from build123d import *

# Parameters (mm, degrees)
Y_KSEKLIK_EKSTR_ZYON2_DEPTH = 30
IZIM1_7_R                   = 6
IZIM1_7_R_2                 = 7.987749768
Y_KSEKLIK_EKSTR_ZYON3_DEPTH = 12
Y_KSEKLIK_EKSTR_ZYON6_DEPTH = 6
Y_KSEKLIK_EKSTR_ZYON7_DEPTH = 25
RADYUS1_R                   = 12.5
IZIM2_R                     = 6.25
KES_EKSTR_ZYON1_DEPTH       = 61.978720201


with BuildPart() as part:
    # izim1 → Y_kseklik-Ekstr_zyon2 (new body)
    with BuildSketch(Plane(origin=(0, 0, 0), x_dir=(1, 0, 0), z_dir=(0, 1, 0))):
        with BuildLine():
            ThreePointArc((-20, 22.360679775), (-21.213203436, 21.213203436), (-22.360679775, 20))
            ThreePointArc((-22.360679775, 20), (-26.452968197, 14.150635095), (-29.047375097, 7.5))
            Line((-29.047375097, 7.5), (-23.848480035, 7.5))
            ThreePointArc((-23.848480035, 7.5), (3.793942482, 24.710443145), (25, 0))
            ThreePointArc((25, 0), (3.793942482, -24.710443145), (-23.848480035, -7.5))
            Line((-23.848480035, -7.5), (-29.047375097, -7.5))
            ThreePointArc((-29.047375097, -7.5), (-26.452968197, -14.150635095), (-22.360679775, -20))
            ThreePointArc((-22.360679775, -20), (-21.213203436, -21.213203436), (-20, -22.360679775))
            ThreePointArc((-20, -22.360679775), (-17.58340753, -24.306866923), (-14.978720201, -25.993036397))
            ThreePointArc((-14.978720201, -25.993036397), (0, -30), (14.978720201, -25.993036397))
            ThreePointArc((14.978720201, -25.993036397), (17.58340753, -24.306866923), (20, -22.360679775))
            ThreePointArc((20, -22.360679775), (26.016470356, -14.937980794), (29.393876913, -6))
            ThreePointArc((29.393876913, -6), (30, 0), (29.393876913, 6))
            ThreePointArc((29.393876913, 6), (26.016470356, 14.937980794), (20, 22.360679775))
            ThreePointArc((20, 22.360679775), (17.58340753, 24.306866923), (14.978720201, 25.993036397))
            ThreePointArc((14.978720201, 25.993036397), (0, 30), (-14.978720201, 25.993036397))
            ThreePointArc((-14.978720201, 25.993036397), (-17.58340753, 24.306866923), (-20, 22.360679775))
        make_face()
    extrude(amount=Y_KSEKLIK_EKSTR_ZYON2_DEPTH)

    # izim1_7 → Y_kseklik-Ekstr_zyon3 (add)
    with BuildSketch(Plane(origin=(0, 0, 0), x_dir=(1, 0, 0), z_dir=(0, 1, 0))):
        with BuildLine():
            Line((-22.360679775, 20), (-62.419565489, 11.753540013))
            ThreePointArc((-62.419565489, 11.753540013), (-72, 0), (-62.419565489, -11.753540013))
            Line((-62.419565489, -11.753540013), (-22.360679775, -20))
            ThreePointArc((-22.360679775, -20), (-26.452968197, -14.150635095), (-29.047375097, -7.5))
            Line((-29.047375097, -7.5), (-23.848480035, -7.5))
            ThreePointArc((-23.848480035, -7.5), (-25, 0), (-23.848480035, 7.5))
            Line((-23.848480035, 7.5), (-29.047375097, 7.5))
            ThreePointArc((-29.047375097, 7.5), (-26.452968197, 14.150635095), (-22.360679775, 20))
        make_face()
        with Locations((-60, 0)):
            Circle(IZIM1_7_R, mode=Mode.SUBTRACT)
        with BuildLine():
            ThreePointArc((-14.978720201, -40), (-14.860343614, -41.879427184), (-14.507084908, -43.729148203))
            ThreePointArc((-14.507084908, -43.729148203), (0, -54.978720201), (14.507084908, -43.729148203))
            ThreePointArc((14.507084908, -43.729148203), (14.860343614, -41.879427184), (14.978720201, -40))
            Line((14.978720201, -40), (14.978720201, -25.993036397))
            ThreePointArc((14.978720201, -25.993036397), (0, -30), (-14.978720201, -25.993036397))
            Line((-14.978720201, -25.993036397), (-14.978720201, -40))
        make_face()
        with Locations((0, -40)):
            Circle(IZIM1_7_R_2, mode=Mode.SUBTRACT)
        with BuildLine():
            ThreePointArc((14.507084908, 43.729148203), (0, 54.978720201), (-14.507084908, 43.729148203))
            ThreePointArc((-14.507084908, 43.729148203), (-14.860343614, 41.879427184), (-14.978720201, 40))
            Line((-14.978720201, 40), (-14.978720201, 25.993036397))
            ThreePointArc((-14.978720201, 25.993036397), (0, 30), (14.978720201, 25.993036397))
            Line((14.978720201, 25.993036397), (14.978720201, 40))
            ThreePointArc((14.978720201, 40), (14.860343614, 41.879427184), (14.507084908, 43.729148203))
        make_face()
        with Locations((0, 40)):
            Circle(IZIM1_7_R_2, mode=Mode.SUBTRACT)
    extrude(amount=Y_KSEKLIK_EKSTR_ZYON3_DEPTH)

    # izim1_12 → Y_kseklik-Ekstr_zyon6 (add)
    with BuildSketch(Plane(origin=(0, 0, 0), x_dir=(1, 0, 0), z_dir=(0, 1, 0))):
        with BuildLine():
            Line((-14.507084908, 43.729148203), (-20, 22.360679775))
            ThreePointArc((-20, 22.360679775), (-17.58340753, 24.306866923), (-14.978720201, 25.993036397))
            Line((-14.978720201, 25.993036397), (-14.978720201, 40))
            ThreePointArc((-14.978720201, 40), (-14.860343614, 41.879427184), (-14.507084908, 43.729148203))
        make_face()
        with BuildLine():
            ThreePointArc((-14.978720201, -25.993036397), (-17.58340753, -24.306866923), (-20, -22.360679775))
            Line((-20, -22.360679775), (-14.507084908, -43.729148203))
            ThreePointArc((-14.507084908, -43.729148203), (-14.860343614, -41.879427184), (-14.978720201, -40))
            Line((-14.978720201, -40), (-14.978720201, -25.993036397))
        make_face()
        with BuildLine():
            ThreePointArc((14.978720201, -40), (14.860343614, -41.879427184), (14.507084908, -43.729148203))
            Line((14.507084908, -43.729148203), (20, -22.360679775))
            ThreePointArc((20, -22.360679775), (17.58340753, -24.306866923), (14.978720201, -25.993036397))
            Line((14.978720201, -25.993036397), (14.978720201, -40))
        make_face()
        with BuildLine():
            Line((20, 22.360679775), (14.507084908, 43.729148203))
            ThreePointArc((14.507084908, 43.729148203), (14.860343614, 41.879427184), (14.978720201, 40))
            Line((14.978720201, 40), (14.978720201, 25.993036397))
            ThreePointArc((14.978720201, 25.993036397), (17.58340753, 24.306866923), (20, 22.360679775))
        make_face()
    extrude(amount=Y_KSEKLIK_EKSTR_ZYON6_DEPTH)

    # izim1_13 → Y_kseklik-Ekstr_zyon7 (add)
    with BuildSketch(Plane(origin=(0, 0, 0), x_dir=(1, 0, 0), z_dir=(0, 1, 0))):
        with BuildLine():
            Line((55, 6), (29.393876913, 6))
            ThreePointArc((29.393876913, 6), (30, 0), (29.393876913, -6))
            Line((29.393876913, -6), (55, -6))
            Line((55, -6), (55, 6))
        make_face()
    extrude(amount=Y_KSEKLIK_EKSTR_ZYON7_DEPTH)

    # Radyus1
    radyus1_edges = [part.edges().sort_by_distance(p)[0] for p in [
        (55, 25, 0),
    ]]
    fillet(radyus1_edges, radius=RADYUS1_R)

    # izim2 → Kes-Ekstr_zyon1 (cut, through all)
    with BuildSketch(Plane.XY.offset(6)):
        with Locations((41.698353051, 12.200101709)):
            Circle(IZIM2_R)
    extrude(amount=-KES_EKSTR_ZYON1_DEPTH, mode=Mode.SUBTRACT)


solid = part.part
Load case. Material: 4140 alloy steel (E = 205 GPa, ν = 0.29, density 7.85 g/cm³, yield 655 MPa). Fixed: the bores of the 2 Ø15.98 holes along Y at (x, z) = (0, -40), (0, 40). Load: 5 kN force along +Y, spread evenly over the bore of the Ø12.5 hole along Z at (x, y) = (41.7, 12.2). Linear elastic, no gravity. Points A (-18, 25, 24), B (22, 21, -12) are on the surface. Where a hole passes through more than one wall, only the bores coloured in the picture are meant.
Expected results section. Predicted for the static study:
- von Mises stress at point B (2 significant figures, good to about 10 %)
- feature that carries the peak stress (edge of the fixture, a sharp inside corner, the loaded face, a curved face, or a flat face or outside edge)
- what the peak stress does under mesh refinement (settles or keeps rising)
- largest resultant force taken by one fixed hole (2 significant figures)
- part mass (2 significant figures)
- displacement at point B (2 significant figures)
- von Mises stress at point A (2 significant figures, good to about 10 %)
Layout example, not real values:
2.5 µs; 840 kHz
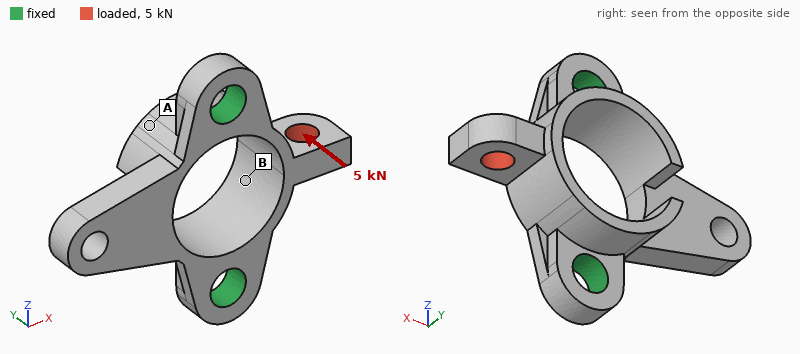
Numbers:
100 MPa; a sharp inside corner; keeps rising; 2.9 kN; 440 g; 0.063 mm; 38 MPa
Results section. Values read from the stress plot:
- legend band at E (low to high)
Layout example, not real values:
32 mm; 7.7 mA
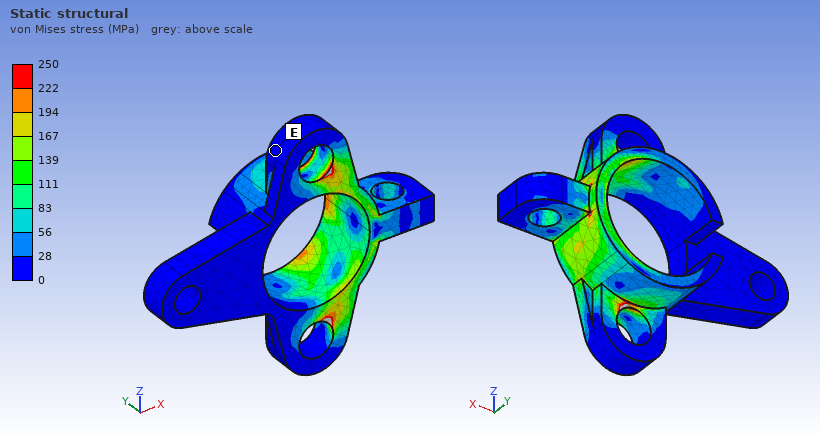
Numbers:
0 to 28 MPa
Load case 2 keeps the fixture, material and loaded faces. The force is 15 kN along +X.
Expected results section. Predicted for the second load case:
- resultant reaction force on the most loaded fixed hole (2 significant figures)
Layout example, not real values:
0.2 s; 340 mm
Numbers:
11 kN
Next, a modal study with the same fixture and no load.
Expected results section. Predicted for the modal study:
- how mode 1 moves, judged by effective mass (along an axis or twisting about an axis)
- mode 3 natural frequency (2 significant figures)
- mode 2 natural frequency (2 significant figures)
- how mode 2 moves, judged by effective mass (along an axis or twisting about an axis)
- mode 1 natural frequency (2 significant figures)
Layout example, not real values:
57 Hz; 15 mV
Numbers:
along Y; 6800 Hz; 3600 Hz; along Y; 2300 Hz
